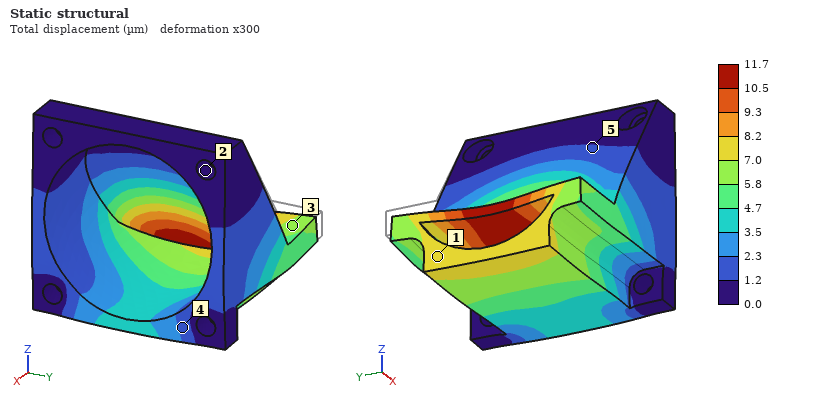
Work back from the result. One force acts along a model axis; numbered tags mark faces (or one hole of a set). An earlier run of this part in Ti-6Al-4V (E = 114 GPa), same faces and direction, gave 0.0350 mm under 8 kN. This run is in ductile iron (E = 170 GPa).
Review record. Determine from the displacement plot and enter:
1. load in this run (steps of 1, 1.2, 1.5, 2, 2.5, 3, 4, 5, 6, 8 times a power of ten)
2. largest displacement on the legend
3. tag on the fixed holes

4 kN
11.7 µm
2
